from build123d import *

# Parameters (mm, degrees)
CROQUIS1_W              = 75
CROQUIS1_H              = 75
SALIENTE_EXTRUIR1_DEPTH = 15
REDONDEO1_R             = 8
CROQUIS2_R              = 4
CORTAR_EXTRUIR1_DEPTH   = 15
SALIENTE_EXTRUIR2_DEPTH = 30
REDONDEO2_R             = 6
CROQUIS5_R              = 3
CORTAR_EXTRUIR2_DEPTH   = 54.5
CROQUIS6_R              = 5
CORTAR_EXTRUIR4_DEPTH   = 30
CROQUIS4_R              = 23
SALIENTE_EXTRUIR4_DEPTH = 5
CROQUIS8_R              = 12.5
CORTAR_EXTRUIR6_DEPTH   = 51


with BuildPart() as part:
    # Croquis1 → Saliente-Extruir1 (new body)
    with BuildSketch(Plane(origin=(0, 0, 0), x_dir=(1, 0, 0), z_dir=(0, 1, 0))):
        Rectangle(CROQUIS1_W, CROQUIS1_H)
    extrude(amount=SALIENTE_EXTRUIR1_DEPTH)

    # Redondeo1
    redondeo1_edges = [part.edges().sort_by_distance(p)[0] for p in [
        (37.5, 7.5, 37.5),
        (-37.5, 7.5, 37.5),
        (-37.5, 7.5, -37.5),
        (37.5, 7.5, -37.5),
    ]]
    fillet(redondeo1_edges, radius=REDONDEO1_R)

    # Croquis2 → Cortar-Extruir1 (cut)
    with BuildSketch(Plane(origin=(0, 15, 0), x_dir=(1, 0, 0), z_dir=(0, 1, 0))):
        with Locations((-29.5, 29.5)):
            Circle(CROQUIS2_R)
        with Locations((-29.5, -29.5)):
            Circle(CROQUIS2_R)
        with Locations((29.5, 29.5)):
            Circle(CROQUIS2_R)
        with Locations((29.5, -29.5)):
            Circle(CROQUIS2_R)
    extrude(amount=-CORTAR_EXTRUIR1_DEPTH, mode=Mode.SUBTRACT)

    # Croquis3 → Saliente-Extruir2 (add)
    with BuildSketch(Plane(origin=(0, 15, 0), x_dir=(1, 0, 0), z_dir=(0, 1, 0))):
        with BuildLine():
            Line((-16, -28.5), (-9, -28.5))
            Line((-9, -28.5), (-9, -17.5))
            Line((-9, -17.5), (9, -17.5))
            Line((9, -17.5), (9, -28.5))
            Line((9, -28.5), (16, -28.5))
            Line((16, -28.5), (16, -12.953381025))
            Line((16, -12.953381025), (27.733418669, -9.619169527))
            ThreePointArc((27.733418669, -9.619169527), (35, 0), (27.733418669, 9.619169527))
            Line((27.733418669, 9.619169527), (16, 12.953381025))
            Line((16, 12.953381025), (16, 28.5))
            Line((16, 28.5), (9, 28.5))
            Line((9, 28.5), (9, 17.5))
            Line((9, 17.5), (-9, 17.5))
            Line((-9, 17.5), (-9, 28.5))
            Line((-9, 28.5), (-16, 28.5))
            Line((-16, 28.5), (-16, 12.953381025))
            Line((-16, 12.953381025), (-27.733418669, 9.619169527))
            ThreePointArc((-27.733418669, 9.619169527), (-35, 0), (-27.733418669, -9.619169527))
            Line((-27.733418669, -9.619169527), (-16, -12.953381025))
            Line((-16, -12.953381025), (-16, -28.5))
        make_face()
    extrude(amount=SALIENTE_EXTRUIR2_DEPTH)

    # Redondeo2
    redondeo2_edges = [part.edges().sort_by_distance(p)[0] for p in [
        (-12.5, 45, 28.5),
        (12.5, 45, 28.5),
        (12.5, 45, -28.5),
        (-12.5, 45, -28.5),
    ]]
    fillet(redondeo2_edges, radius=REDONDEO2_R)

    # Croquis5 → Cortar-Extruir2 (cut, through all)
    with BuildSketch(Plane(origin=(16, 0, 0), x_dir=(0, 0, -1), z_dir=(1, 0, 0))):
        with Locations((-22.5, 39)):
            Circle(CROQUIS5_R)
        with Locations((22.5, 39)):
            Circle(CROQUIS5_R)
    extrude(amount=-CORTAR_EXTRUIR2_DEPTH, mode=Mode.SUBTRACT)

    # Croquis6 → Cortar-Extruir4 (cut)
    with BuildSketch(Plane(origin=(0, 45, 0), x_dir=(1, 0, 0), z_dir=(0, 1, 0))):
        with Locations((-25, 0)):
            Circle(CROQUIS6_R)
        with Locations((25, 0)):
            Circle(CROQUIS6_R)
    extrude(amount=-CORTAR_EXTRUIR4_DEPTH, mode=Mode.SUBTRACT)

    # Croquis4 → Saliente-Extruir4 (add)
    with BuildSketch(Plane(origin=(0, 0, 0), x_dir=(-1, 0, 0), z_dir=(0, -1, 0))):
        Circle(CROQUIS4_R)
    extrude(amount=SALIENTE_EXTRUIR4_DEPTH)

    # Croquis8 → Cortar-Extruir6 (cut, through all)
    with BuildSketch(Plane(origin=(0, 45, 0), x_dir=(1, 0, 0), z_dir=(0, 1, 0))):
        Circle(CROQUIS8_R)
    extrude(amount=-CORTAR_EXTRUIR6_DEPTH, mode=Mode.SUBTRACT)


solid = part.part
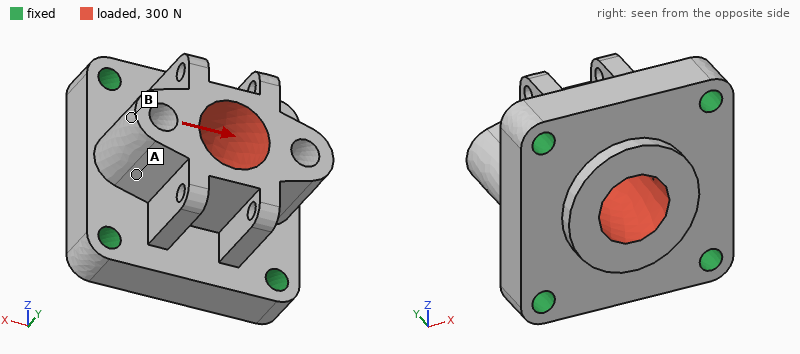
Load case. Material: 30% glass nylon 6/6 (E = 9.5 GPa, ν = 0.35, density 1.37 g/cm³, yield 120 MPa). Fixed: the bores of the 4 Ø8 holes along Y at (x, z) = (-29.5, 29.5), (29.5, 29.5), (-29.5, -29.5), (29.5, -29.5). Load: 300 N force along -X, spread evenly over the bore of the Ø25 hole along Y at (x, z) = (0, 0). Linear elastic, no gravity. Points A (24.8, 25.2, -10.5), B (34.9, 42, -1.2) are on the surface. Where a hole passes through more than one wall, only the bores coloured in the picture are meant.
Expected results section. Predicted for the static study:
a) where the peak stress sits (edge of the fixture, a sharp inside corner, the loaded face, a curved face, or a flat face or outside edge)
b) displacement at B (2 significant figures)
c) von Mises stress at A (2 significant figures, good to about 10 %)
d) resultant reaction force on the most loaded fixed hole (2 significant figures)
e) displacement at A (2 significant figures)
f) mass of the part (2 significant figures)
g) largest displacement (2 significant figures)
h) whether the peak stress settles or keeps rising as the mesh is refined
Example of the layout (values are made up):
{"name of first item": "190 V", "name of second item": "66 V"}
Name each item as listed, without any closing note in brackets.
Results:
{"where the peak stress sits": "edge of the fixture", "displacement at B": "3.2 µm", "von Mises stress at A": "0.16 MPa", "resultant reaction force on the most loaded fixed hole": "89 N", "displacement at A": "2.1 µm", "mass of the part": "170 g", "largest displacement": "3.3 µm", "whether the peak stress settles or keeps rising as the mesh is refined": "keeps rising"}
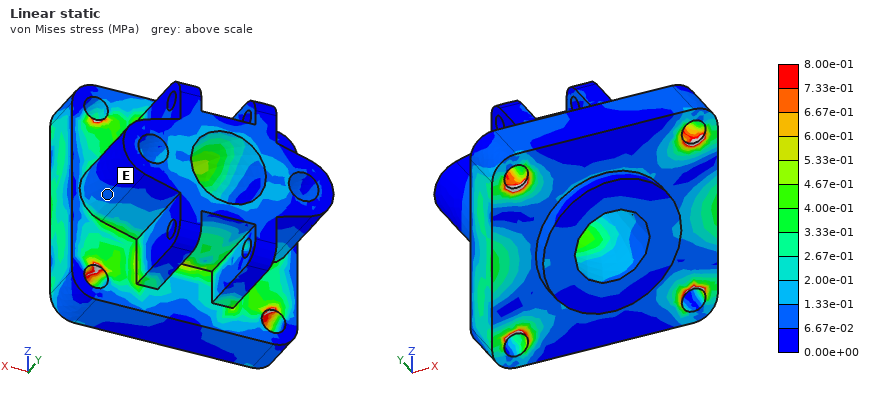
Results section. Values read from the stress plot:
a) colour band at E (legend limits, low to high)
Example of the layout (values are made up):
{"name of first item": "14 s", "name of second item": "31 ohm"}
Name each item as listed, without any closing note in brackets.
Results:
{"colour band at E": "6.67e-02 to 1.33e-01 MPa"}
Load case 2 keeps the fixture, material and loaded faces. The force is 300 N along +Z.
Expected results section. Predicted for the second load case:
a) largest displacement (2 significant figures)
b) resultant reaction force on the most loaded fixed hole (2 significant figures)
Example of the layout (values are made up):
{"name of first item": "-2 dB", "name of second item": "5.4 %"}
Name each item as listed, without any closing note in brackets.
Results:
{"largest displacement": "3.2 µm", "resultant reaction force on the most loaded fixed hole": "89 N"}
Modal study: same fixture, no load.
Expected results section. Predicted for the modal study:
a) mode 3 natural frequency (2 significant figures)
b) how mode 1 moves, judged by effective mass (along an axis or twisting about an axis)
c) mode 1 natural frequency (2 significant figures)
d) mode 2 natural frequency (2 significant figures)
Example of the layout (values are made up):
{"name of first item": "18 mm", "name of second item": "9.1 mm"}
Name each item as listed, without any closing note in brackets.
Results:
{"mode 3 natural frequency": "5800 Hz", "how mode 1 moves, judged by effective mass": "along X", "mode 1 natural frequency": "5200 Hz", "mode 2 natural frequency": "5700 Hz"}
